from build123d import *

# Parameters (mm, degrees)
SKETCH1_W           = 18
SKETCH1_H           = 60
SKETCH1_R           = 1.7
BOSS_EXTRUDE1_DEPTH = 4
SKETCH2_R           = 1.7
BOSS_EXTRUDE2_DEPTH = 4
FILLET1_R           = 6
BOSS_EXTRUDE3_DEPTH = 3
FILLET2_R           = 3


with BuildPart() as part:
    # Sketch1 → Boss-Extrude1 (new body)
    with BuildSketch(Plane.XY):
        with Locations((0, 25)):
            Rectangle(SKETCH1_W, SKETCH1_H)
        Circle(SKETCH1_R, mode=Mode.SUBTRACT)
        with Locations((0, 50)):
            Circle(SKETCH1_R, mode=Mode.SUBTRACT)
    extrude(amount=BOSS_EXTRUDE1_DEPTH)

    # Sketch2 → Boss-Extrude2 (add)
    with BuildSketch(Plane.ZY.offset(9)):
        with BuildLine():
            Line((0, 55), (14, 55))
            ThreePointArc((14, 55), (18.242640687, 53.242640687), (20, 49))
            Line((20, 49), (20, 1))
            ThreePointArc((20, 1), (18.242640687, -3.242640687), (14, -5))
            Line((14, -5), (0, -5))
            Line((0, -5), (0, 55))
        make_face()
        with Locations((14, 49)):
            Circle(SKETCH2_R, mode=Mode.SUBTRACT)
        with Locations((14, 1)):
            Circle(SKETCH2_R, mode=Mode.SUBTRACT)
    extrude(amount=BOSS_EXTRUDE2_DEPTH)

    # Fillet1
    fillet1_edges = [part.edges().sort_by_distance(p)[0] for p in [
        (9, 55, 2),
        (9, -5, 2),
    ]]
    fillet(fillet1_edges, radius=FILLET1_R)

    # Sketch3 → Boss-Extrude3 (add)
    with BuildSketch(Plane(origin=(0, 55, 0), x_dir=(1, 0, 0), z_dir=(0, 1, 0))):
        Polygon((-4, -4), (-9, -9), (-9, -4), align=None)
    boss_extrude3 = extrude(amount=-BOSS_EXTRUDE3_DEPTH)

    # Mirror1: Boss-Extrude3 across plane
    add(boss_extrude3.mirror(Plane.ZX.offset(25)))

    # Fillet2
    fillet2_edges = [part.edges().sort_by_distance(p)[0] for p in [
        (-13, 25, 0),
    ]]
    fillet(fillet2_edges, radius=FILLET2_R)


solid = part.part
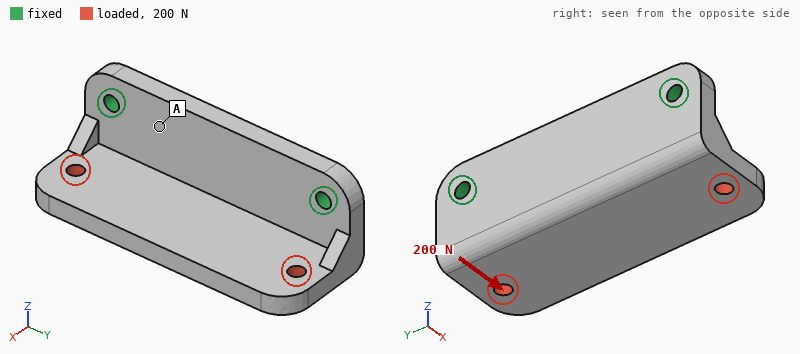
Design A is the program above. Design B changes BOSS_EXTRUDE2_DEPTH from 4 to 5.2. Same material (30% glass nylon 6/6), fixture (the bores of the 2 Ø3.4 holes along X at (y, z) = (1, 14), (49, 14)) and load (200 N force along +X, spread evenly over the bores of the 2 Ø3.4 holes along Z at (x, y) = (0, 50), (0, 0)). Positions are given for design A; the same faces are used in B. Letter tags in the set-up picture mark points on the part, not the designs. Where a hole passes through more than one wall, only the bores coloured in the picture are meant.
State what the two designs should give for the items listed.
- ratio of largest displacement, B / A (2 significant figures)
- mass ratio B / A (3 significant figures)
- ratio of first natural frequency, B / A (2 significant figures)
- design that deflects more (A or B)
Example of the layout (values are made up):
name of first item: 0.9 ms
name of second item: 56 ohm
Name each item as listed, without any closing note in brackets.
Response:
ratio of largest displacement, B / A: 0.53
mass ratio B / A: 1.16
ratio of first natural frequency, B / A: 1.3
design that deflects more: A
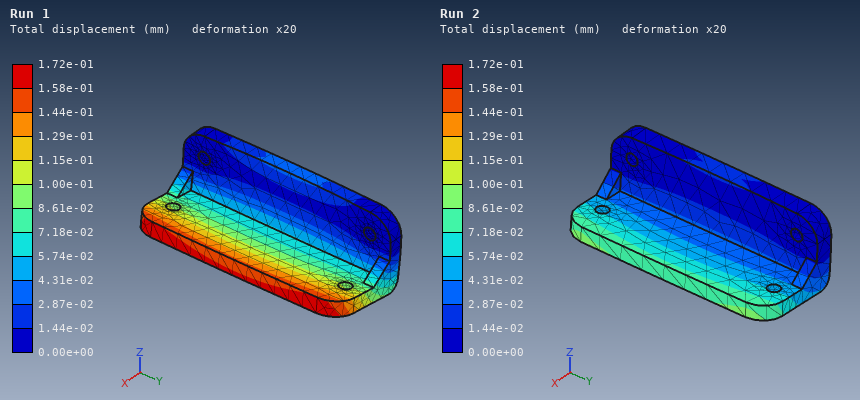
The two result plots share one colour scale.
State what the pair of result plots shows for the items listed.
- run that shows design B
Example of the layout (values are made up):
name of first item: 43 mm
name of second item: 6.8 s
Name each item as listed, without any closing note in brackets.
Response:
run that shows design B: Run 2
